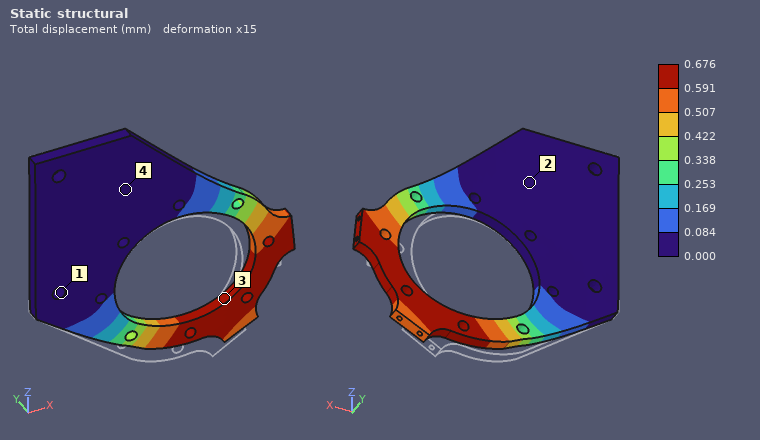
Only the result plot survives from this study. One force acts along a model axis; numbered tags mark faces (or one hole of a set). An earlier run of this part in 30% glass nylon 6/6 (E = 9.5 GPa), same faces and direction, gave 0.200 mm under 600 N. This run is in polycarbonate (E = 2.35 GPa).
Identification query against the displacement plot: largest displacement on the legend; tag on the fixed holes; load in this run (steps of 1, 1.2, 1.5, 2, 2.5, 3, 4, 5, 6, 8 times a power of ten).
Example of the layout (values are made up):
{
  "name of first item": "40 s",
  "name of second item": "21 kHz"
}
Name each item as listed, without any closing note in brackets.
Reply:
{
  "largest displacement on the legend": "0.676 mm",
  "tag on the fixed holes": "1",
  "load in this run": "500 N"
}
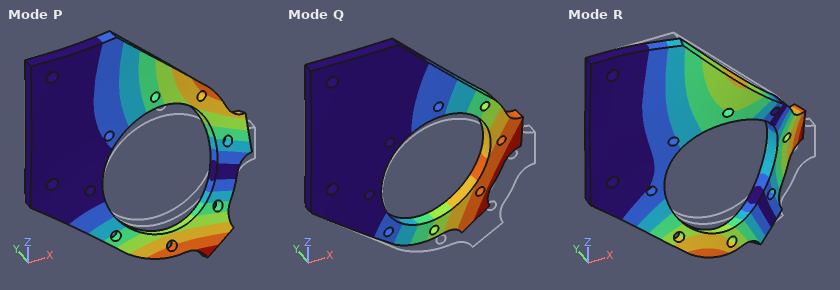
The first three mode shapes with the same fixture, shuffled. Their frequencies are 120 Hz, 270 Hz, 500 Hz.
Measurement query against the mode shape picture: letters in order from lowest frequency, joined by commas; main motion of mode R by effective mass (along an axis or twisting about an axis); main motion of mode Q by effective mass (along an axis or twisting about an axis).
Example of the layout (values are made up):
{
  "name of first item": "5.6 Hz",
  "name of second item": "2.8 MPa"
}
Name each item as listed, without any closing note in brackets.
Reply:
{
  "letters in order from lowest frequency, joined by commas": "Q, P, R",
  "main motion of mode R by effective mass": "along Y",
  "main motion of mode Q by effective mass": "along Y"
}
